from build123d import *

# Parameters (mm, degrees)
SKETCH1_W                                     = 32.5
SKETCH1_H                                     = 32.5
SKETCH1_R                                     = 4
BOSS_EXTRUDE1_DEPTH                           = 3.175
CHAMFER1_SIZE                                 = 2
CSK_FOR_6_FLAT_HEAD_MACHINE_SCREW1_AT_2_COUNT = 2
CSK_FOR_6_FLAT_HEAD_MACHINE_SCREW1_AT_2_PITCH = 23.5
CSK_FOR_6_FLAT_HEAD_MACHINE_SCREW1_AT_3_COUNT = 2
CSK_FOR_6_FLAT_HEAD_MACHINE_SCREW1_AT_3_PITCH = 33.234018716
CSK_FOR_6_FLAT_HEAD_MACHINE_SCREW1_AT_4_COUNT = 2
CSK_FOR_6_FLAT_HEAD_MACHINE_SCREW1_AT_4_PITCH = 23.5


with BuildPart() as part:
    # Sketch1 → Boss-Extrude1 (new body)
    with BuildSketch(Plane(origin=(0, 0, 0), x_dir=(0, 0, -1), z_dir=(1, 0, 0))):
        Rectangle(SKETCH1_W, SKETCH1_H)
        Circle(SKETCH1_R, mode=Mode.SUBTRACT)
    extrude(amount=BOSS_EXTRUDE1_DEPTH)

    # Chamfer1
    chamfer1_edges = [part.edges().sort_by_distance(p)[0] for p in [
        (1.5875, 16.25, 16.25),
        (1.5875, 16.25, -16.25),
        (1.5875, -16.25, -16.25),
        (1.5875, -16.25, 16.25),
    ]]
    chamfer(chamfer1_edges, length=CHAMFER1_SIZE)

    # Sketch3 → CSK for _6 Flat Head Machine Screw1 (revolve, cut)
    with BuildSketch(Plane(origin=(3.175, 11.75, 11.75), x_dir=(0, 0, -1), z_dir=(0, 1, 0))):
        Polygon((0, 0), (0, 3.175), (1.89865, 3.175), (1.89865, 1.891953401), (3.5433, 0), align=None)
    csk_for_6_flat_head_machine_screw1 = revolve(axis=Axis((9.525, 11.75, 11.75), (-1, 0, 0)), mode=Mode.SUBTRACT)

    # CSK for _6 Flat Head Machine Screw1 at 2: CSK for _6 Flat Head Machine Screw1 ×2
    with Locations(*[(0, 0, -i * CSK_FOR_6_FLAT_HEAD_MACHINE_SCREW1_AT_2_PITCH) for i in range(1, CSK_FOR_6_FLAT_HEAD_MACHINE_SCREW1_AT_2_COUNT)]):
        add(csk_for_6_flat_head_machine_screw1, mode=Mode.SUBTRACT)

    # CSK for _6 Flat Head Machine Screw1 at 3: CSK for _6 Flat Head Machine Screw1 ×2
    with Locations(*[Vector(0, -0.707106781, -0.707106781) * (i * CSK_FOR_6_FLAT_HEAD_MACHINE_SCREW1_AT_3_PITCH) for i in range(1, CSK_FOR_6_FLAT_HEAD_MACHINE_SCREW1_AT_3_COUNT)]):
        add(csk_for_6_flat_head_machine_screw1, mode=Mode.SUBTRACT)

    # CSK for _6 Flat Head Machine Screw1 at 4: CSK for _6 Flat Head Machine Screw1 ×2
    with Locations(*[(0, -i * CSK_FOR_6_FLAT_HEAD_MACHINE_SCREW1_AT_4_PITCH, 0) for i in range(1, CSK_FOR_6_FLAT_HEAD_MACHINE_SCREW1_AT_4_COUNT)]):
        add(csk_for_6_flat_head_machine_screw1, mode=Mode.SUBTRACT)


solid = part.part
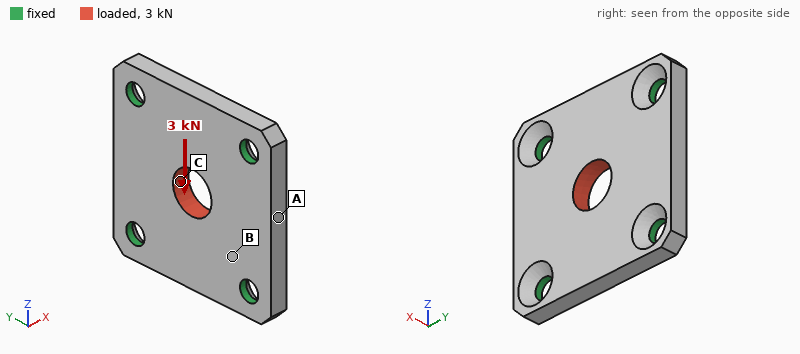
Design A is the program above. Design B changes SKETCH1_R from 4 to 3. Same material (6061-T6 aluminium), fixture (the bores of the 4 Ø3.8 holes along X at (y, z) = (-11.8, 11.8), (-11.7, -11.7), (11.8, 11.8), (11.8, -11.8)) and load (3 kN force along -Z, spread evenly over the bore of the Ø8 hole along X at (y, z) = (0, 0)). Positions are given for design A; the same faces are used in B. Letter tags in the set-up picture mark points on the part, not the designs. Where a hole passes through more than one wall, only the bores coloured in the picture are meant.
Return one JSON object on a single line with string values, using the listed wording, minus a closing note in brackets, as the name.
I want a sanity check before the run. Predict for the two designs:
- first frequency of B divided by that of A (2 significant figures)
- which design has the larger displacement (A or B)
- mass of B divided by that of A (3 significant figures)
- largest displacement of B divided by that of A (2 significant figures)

{"first frequency of B divided by that of A": "0.98", "which design has the larger displacement": "B", "mass of B divided by that of A": "1.02", "largest displacement of B divided by that of A": "1.1"}
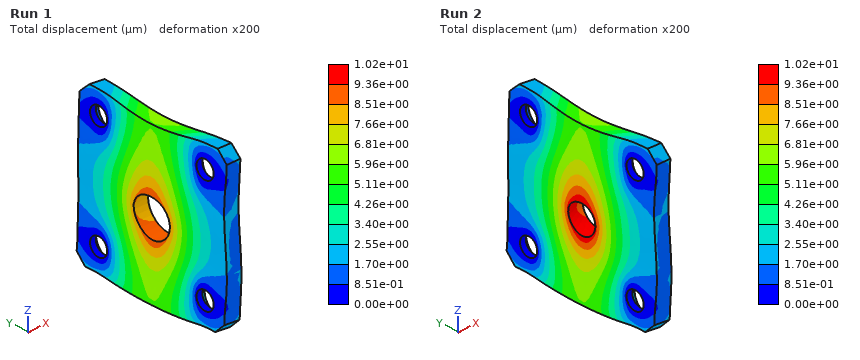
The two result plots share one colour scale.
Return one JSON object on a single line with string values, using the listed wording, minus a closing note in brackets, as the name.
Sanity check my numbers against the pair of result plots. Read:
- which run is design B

{"which run is design B": "Run 2"}
